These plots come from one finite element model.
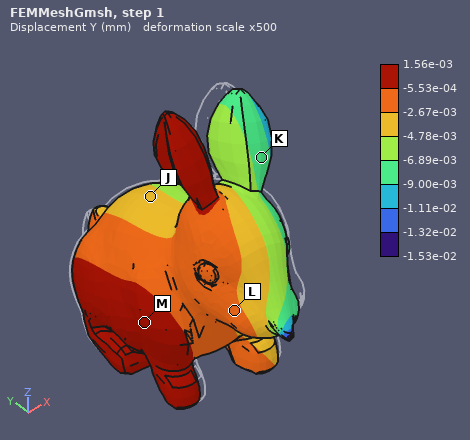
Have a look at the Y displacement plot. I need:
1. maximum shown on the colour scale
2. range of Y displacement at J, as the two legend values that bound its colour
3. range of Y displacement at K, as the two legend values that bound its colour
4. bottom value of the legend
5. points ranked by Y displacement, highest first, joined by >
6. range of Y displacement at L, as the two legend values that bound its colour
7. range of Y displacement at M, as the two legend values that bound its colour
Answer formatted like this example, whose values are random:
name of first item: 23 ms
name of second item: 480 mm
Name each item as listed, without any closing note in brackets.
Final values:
maximum shown on the colour scale: 1.56e-03 mm
range of Y displacement at J, as the two legend values that bound its colour: -4.78e-03 to -2.67e-03 mm
range of Y displacement at K, as the two legend values that bound its colour: -9.00e-03 to -6.89e-03 mm
bottom value of the legend: -1.53e-02 mm
points ranked by Y displacement, highest first, joined by >: M > L > J > K
range of Y displacement at L, as the two legend values that bound its colour: -2.67e-03 to -5.53e-04 mm
range of Y displacement at M, as the two legend values that bound its colour: -5.53e-04 to 1.56e-03 mm
